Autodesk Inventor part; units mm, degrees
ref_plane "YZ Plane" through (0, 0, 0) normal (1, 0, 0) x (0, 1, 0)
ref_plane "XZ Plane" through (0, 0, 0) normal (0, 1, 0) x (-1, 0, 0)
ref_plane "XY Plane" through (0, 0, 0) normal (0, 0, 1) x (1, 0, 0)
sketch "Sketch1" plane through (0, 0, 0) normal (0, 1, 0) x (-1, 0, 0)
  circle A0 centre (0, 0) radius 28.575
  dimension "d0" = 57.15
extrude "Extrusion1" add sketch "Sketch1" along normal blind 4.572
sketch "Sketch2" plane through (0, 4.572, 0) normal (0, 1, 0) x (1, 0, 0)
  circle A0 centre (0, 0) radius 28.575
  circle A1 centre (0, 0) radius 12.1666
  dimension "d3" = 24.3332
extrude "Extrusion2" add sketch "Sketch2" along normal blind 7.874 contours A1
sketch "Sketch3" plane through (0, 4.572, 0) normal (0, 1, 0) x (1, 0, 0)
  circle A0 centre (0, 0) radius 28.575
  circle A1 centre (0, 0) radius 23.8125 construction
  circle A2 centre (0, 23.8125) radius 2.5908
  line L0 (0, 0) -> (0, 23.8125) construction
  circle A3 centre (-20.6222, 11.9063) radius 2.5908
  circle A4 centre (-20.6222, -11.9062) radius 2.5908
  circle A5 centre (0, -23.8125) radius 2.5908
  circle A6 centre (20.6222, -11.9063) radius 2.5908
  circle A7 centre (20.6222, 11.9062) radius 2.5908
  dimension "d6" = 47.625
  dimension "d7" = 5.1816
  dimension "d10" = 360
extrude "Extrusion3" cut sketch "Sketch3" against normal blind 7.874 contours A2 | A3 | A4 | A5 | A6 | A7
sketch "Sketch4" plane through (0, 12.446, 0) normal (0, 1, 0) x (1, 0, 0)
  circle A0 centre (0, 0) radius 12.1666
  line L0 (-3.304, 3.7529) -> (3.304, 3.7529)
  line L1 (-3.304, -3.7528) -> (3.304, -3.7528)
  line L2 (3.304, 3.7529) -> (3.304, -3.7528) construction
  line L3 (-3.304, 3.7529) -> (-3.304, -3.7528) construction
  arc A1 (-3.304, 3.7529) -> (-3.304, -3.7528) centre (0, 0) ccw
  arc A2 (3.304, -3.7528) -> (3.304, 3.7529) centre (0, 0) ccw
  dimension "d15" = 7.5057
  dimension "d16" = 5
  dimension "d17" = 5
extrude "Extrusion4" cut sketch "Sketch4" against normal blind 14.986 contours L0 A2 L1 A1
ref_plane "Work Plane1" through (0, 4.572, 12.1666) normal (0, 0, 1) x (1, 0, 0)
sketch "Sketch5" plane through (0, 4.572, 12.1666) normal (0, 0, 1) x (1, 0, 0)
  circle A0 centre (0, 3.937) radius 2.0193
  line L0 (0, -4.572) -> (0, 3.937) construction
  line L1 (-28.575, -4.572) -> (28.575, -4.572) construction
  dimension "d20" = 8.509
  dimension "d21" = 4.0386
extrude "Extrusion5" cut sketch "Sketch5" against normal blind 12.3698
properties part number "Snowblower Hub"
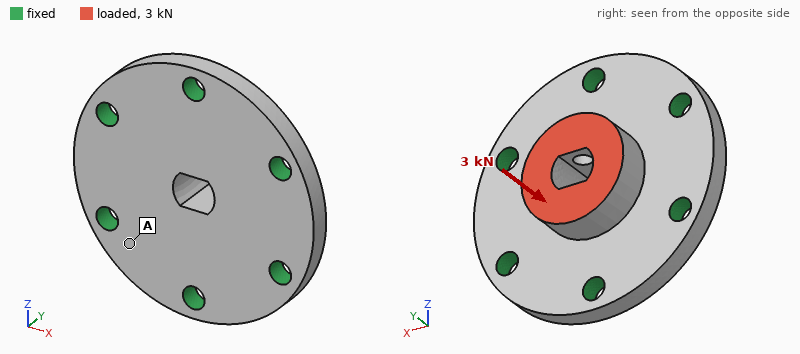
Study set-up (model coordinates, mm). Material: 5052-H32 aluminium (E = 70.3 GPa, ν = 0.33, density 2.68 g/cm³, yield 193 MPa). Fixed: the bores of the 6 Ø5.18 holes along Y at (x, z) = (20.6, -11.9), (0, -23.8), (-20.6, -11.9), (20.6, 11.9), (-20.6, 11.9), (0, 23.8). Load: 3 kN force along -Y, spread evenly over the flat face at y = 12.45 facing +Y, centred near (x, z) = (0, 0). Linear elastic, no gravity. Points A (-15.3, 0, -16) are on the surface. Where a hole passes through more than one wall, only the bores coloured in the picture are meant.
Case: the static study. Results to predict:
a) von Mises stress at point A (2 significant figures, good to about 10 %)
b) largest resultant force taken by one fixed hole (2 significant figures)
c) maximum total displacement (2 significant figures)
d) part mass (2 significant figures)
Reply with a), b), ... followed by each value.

a) 18 MPa
b) 550 N
c) 17 µm
d) 37 g
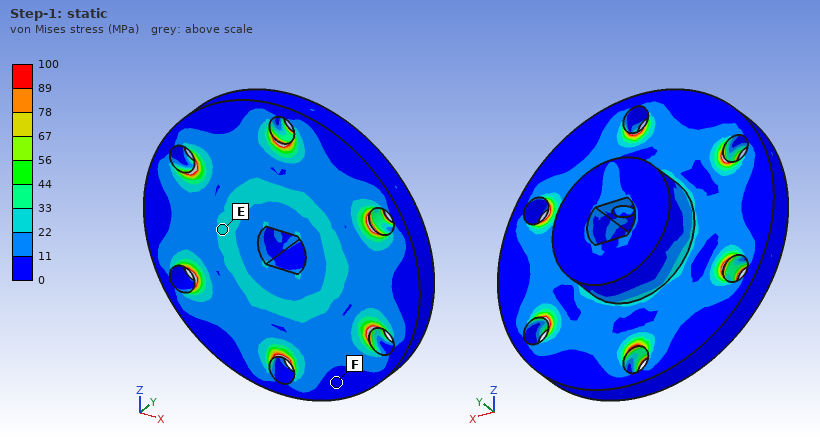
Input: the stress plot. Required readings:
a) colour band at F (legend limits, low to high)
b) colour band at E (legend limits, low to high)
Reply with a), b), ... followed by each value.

a) 0 to 11 MPa
b) 22 to 33 MPa
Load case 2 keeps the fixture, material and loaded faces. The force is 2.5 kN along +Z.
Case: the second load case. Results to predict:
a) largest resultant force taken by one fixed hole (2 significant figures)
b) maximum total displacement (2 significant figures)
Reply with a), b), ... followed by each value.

a) 790 N
b) 17 µm
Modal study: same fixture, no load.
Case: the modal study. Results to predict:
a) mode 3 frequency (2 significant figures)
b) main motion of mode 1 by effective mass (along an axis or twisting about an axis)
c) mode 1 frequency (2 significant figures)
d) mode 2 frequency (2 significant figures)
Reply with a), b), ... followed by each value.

a) 26 kHz
b) along Y
c) 18 kHz
d) 26 kHz
